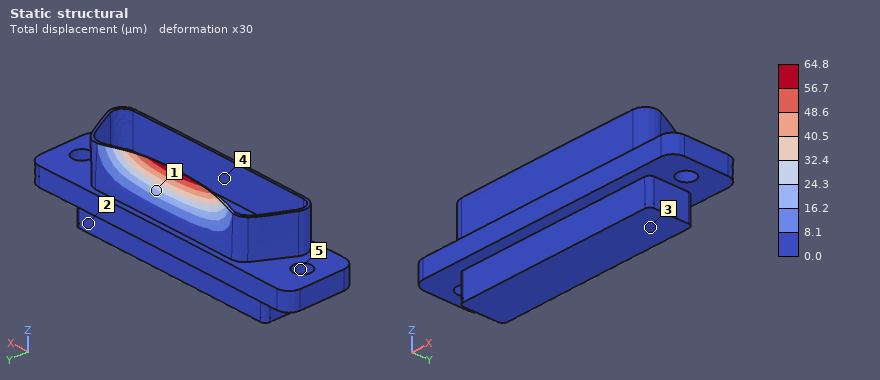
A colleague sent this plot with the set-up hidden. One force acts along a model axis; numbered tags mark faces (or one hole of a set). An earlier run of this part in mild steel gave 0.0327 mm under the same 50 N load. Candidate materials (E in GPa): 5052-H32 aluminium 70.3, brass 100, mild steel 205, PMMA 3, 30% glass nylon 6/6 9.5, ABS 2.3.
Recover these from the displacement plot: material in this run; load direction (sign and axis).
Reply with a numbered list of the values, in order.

1. brass
2. -Y
